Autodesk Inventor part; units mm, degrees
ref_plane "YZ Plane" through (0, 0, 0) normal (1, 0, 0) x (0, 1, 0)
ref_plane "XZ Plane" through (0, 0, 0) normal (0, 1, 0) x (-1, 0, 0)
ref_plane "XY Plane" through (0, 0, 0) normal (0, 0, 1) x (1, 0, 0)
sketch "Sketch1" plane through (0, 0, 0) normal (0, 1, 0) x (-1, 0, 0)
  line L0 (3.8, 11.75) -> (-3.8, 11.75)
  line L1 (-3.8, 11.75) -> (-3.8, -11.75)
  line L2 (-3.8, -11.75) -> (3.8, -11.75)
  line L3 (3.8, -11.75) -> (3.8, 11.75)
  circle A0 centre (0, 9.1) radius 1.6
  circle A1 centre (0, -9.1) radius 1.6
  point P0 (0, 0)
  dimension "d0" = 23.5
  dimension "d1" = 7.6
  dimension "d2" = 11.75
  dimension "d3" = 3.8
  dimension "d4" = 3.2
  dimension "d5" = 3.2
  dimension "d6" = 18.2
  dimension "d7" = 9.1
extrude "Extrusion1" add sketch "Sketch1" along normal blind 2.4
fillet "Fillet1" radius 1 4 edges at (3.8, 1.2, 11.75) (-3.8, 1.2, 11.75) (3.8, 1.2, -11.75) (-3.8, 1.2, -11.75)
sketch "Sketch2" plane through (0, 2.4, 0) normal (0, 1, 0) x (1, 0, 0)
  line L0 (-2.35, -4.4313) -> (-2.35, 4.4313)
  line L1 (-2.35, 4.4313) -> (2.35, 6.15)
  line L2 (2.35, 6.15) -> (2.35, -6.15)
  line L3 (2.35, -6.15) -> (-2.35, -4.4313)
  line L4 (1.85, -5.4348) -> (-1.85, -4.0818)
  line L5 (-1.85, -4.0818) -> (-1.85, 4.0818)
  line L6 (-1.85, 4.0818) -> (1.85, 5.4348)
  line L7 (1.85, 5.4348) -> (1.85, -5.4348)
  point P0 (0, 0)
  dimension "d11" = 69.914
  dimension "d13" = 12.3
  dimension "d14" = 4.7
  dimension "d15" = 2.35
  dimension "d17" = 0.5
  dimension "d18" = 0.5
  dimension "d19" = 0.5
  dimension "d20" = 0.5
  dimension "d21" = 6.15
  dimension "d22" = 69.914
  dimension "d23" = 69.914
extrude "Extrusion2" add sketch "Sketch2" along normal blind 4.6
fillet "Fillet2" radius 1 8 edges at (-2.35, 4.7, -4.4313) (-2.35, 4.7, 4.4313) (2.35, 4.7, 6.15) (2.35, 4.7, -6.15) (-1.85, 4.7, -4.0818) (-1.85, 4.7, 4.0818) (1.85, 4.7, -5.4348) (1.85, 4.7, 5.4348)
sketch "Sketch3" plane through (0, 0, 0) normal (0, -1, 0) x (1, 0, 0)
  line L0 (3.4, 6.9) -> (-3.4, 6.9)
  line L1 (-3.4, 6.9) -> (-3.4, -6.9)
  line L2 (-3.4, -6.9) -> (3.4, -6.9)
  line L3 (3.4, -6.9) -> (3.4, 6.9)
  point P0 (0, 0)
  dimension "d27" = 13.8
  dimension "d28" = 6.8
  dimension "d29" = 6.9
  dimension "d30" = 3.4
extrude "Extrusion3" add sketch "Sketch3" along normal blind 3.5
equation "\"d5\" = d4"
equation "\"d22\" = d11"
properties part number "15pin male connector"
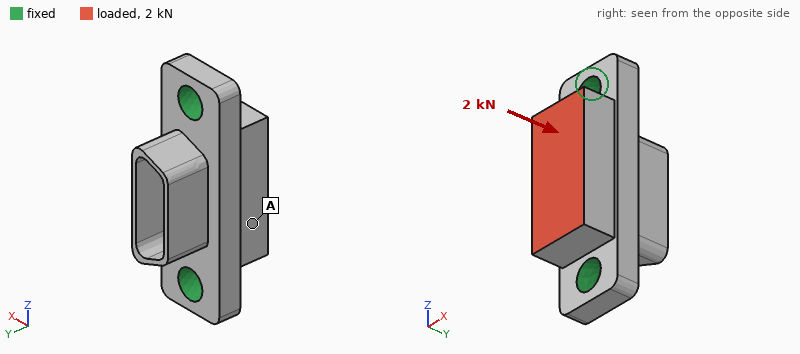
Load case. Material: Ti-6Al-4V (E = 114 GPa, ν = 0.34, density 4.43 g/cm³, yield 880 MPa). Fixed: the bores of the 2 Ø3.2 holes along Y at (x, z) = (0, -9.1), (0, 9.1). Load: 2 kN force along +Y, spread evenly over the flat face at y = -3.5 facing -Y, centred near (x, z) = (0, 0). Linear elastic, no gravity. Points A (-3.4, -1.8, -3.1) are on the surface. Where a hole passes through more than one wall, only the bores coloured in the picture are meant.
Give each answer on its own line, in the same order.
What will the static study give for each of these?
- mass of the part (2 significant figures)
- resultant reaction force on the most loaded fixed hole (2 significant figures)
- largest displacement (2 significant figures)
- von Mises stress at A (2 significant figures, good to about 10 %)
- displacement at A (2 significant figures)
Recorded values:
3.5 g
1.1 kN
8.7 µm
38 MPa
7.6 µm
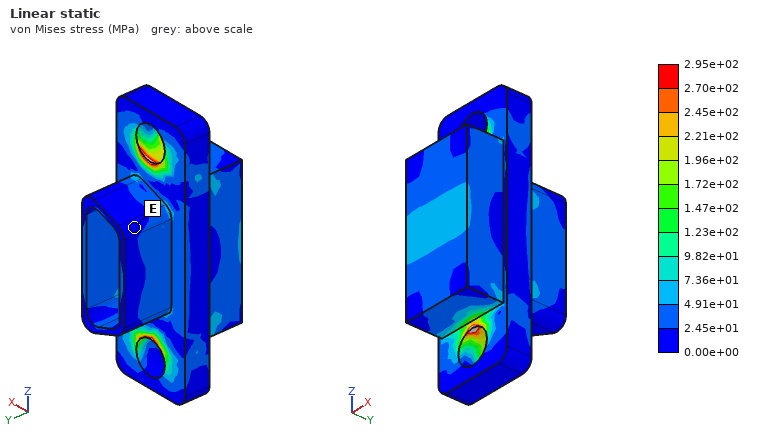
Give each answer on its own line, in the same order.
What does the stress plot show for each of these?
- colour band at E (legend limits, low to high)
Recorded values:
0.00e+00 to 2.45e+01 MPa
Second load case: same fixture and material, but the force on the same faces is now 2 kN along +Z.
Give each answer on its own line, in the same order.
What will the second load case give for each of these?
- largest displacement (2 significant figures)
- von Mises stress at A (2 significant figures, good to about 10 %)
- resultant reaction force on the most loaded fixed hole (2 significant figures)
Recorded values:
6.7 µm
48 MPa
1.2 kN
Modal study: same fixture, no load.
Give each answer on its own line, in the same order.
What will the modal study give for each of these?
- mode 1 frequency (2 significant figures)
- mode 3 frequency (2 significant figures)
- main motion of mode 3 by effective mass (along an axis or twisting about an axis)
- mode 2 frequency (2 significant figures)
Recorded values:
32 kHz
41 kHz
along X
36 kHz
